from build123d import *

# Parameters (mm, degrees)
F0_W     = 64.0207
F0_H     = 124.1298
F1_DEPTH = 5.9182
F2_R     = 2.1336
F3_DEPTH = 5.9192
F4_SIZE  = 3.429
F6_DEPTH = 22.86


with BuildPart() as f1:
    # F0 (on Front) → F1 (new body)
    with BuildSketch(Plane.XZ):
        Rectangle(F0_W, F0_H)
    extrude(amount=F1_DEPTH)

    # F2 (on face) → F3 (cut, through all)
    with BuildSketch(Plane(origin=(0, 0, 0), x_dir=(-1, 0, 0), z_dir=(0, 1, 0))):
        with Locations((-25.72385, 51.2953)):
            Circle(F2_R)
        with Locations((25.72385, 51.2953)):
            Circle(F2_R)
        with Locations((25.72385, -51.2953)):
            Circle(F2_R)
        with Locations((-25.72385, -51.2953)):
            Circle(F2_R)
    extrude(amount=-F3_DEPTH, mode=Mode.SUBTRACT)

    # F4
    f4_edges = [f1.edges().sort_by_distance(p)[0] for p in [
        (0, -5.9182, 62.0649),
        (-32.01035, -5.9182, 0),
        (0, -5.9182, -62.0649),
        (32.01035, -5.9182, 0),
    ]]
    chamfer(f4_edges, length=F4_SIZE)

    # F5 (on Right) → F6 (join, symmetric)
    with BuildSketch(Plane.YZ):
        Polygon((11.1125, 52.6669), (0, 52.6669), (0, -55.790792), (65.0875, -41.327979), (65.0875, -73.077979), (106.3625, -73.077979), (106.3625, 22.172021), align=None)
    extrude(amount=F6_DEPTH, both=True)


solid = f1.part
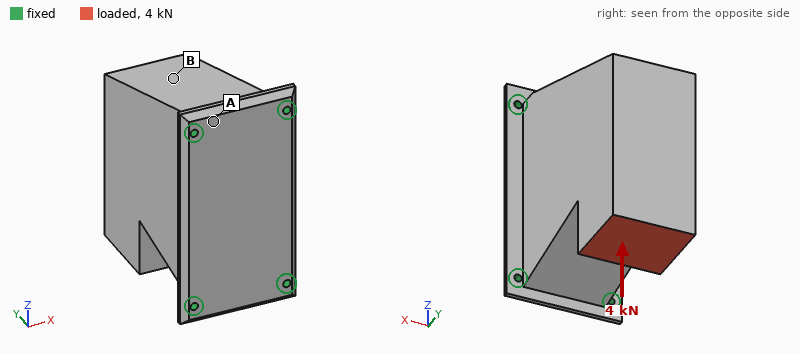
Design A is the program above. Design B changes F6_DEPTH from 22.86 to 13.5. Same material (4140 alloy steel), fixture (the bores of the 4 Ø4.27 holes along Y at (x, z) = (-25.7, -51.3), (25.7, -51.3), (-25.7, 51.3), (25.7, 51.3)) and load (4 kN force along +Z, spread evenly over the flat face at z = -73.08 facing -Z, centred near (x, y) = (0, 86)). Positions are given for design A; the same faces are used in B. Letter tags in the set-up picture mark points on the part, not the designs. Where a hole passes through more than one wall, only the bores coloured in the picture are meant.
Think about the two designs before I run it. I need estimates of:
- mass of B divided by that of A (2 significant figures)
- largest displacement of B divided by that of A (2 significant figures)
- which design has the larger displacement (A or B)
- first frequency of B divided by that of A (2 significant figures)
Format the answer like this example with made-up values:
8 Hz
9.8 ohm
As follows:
0.63
3.2
B
0.60
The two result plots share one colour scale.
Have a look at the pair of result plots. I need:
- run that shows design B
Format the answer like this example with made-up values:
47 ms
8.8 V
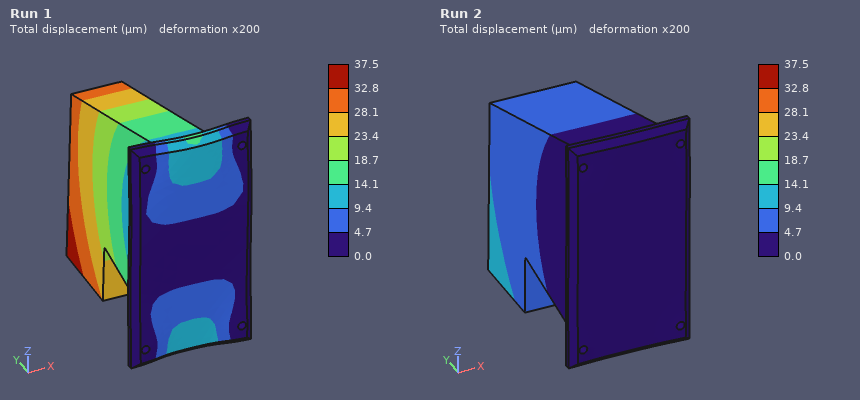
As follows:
Run 1
